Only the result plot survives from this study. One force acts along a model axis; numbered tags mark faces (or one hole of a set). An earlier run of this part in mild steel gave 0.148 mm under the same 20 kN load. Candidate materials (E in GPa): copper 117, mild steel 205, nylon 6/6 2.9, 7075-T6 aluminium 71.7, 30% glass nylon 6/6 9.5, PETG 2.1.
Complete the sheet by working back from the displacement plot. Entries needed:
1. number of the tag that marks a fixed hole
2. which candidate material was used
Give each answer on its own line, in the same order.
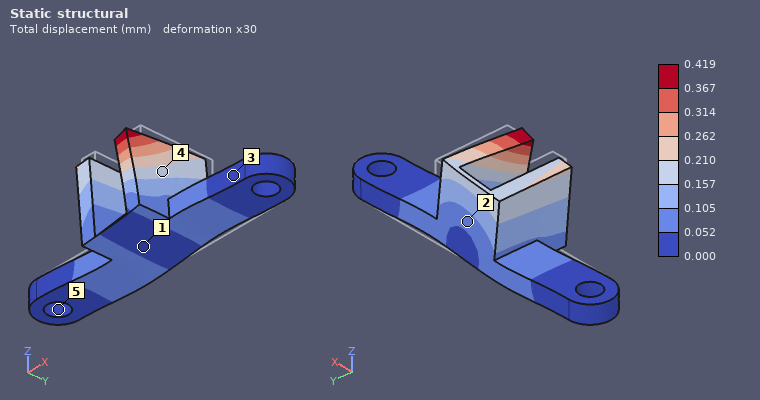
5
7075-T6 aluminium
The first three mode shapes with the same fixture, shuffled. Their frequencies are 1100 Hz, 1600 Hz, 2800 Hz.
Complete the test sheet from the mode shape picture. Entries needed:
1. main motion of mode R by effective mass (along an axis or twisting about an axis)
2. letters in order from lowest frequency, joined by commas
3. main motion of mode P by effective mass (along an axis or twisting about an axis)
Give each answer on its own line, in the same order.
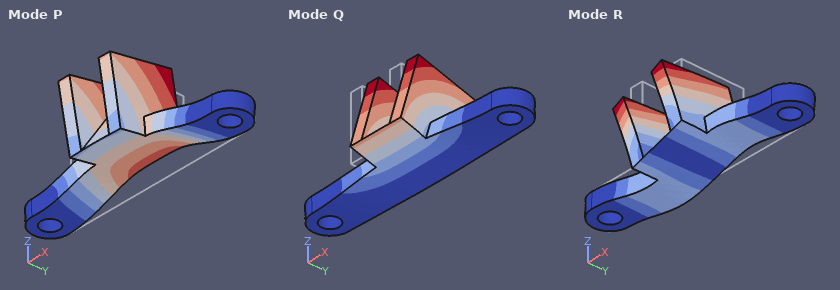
along X
Q, P, R
along Z
